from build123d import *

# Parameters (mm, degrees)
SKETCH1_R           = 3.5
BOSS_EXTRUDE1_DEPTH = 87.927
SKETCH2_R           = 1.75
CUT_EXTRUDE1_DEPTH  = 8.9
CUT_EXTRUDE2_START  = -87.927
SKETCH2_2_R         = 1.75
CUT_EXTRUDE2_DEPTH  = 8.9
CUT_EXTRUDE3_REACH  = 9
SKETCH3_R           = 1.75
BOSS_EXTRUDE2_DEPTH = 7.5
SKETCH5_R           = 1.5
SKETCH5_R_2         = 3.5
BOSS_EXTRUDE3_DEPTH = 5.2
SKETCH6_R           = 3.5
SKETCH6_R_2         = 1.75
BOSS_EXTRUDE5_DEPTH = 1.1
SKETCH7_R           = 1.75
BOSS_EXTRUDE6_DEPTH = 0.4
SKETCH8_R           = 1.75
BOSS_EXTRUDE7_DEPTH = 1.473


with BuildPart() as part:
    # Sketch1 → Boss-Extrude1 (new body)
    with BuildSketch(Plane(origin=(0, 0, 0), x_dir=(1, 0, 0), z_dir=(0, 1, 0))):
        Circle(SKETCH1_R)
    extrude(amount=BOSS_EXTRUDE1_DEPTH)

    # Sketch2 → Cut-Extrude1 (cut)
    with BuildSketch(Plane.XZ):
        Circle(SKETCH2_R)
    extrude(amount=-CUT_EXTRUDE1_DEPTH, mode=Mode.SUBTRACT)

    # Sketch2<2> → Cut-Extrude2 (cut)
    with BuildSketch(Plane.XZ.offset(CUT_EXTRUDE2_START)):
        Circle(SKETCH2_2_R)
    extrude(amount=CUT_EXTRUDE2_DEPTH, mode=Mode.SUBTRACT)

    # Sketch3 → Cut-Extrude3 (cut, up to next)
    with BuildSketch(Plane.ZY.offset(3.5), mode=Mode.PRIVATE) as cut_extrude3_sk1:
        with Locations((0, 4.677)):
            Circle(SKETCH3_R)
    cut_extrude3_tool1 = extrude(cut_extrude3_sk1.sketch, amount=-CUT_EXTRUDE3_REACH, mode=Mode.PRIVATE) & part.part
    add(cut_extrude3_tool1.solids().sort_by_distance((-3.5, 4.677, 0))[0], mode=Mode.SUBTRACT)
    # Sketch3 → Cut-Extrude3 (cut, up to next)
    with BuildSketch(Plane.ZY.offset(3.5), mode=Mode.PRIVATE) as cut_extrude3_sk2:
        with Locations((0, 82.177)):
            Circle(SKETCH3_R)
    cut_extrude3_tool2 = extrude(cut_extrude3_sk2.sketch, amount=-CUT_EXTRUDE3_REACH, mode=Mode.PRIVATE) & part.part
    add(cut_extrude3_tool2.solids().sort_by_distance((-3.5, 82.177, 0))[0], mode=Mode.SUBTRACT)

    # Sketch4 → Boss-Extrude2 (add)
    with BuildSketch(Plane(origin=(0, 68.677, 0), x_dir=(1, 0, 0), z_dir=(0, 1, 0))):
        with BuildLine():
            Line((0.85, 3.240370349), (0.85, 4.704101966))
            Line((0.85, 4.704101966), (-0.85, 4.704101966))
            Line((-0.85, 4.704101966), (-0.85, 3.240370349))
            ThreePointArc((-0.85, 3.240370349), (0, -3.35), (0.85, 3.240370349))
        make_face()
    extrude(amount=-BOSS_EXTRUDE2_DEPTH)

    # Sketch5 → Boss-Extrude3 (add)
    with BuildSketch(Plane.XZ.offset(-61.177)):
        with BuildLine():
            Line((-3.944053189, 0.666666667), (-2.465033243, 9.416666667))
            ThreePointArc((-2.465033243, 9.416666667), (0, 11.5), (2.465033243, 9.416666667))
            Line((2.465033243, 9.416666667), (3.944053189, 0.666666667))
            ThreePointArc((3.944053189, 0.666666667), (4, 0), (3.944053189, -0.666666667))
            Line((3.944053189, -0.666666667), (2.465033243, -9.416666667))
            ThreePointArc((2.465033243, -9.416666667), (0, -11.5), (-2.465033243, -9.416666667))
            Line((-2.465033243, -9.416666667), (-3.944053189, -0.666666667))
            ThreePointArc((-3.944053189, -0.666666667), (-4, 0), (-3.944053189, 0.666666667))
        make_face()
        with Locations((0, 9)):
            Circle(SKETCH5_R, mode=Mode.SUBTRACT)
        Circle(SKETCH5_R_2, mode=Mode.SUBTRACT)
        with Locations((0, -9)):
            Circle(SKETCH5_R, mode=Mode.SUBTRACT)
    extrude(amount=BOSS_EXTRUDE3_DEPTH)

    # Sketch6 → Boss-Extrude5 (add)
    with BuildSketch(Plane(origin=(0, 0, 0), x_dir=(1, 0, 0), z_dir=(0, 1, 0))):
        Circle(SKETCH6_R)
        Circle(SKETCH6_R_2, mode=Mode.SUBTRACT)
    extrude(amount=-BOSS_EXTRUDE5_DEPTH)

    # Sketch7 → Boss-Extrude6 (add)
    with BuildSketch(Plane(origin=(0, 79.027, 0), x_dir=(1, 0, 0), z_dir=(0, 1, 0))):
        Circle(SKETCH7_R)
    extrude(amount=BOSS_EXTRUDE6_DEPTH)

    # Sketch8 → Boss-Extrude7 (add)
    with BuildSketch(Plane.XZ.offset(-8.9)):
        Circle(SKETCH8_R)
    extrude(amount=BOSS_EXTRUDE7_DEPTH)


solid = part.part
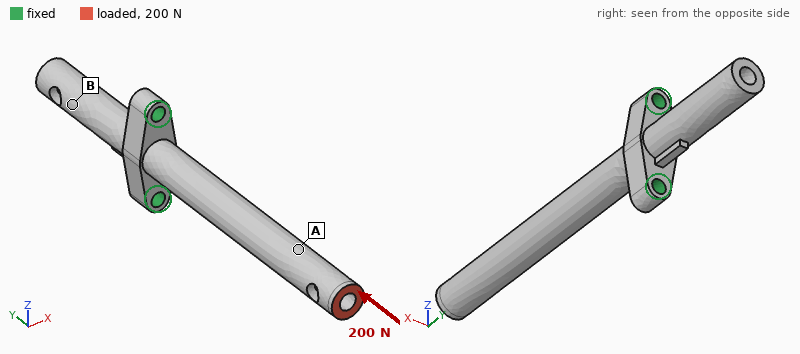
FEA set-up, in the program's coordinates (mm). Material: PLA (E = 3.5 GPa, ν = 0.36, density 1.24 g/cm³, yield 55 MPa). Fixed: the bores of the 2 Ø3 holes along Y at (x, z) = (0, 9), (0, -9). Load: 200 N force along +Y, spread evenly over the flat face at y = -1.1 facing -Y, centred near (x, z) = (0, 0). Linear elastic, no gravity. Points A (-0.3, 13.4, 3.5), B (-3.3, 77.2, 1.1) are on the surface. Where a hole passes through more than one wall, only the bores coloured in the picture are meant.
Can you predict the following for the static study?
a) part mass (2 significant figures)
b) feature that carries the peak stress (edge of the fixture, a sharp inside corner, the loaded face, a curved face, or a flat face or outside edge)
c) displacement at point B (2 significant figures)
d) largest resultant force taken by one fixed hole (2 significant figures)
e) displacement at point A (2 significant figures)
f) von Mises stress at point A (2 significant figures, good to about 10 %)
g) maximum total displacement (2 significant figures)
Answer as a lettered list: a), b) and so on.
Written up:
a) 4.6 g
b) a curved face
c) 0.021 mm
d) 100 N
e) 0.086 mm
f) 5.4 MPa
g) 0.14 mm
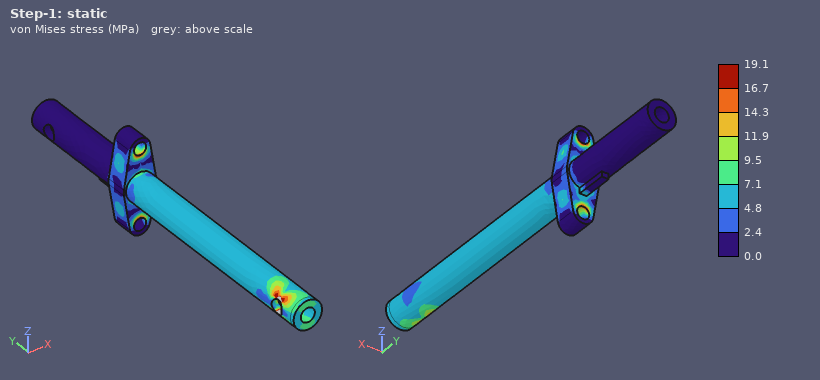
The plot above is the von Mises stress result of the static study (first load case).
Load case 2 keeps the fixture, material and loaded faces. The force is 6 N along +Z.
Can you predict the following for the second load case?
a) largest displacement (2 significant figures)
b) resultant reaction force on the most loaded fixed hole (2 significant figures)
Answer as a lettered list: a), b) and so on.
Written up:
a) 1.0 mm
b) 27 N
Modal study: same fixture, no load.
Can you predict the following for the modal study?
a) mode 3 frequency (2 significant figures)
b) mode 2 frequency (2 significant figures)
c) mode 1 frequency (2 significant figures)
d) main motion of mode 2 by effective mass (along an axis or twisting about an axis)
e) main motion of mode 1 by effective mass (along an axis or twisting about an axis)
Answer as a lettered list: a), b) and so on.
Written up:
a) 1700 Hz
b) 500 Hz
c) 430 Hz
d) along Z
e) along X
